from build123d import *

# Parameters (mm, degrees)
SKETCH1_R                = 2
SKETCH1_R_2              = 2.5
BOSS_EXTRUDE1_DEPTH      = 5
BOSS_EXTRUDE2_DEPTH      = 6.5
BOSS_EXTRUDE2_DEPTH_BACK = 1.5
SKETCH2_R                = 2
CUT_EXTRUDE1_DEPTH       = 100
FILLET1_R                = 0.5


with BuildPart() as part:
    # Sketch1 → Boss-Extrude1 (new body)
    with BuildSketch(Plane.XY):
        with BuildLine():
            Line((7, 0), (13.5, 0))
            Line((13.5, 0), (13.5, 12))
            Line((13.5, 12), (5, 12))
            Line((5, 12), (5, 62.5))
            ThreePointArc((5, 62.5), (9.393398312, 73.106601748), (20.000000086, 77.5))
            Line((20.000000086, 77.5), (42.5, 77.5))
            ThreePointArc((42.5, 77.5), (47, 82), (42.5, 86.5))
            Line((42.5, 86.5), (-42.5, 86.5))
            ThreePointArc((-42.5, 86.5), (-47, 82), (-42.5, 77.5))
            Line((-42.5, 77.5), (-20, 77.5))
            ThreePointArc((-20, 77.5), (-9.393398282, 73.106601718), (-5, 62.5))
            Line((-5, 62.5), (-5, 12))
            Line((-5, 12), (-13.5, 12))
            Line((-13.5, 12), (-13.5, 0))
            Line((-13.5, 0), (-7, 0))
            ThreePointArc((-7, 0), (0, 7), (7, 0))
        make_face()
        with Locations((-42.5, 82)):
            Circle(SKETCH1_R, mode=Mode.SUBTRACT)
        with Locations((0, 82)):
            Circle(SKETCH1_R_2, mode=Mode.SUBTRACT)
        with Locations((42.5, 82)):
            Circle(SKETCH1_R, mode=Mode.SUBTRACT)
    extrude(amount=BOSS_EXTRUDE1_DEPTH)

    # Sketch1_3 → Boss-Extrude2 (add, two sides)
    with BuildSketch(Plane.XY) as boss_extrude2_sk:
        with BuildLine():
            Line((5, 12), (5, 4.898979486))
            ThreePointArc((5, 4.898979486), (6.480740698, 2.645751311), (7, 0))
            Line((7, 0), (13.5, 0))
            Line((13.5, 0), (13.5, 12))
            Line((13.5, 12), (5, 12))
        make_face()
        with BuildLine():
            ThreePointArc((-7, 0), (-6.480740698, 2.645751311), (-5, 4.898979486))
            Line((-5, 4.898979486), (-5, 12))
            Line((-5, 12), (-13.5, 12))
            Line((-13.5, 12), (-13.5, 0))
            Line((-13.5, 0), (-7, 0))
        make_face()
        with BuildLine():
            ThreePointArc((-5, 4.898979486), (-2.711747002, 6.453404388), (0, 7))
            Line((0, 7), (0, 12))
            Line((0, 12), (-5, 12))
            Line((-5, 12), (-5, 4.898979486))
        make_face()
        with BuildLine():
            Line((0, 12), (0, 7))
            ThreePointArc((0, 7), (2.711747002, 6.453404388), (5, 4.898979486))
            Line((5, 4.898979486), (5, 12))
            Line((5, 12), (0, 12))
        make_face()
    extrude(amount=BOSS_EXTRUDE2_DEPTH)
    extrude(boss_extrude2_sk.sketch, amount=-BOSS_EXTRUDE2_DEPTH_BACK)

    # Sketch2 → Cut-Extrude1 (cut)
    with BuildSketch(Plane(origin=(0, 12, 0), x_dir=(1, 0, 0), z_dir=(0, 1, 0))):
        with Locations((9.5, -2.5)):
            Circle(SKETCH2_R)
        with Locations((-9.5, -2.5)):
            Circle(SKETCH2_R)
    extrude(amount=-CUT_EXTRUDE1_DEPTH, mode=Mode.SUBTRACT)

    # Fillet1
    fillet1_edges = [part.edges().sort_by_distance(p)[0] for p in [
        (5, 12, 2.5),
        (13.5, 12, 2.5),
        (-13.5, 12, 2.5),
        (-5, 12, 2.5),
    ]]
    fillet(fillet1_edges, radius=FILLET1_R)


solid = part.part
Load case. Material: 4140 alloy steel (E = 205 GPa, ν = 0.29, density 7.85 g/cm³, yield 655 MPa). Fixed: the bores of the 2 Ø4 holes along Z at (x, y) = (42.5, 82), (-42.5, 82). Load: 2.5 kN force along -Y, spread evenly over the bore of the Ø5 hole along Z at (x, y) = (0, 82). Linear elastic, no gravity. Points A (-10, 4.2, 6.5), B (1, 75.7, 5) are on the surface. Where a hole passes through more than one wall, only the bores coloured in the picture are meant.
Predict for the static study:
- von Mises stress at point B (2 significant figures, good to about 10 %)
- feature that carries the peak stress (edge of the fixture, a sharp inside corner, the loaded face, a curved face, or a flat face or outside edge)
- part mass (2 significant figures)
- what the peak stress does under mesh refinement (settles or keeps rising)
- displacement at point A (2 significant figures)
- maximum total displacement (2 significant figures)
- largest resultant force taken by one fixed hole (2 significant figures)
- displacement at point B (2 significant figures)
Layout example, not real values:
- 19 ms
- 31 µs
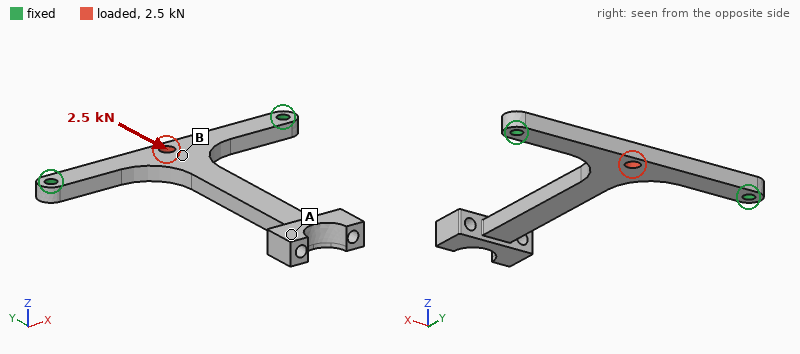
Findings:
- 86 MPa
- edge of the fixture
- 73 g
- keeps rising
- 84 µm
- 89 µm
- 1.5 kN
- 86 µm
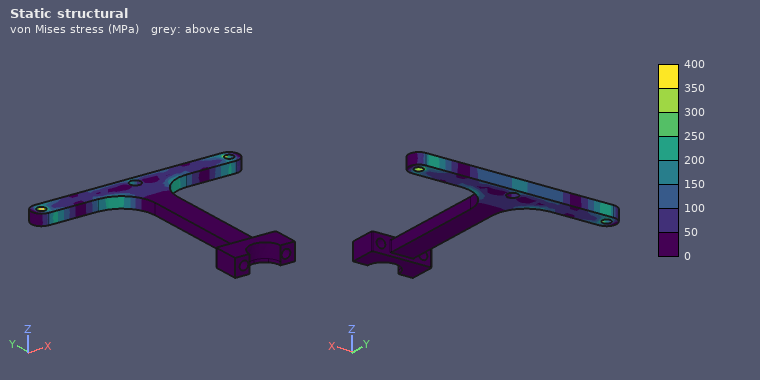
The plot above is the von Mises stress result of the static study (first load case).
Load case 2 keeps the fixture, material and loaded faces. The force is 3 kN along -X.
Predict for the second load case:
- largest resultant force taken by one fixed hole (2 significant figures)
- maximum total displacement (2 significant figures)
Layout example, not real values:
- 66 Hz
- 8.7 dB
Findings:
- 1.5 kN
- 6.9 µm
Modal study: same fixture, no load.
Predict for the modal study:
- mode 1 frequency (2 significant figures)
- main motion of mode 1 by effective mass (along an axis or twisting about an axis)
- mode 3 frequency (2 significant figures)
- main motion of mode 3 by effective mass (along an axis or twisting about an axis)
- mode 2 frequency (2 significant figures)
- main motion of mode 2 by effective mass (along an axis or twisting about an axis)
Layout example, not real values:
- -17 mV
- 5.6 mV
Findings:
- 370 Hz
- along Z
- 2300 Hz
- along Z
- 1100 Hz
- along X
